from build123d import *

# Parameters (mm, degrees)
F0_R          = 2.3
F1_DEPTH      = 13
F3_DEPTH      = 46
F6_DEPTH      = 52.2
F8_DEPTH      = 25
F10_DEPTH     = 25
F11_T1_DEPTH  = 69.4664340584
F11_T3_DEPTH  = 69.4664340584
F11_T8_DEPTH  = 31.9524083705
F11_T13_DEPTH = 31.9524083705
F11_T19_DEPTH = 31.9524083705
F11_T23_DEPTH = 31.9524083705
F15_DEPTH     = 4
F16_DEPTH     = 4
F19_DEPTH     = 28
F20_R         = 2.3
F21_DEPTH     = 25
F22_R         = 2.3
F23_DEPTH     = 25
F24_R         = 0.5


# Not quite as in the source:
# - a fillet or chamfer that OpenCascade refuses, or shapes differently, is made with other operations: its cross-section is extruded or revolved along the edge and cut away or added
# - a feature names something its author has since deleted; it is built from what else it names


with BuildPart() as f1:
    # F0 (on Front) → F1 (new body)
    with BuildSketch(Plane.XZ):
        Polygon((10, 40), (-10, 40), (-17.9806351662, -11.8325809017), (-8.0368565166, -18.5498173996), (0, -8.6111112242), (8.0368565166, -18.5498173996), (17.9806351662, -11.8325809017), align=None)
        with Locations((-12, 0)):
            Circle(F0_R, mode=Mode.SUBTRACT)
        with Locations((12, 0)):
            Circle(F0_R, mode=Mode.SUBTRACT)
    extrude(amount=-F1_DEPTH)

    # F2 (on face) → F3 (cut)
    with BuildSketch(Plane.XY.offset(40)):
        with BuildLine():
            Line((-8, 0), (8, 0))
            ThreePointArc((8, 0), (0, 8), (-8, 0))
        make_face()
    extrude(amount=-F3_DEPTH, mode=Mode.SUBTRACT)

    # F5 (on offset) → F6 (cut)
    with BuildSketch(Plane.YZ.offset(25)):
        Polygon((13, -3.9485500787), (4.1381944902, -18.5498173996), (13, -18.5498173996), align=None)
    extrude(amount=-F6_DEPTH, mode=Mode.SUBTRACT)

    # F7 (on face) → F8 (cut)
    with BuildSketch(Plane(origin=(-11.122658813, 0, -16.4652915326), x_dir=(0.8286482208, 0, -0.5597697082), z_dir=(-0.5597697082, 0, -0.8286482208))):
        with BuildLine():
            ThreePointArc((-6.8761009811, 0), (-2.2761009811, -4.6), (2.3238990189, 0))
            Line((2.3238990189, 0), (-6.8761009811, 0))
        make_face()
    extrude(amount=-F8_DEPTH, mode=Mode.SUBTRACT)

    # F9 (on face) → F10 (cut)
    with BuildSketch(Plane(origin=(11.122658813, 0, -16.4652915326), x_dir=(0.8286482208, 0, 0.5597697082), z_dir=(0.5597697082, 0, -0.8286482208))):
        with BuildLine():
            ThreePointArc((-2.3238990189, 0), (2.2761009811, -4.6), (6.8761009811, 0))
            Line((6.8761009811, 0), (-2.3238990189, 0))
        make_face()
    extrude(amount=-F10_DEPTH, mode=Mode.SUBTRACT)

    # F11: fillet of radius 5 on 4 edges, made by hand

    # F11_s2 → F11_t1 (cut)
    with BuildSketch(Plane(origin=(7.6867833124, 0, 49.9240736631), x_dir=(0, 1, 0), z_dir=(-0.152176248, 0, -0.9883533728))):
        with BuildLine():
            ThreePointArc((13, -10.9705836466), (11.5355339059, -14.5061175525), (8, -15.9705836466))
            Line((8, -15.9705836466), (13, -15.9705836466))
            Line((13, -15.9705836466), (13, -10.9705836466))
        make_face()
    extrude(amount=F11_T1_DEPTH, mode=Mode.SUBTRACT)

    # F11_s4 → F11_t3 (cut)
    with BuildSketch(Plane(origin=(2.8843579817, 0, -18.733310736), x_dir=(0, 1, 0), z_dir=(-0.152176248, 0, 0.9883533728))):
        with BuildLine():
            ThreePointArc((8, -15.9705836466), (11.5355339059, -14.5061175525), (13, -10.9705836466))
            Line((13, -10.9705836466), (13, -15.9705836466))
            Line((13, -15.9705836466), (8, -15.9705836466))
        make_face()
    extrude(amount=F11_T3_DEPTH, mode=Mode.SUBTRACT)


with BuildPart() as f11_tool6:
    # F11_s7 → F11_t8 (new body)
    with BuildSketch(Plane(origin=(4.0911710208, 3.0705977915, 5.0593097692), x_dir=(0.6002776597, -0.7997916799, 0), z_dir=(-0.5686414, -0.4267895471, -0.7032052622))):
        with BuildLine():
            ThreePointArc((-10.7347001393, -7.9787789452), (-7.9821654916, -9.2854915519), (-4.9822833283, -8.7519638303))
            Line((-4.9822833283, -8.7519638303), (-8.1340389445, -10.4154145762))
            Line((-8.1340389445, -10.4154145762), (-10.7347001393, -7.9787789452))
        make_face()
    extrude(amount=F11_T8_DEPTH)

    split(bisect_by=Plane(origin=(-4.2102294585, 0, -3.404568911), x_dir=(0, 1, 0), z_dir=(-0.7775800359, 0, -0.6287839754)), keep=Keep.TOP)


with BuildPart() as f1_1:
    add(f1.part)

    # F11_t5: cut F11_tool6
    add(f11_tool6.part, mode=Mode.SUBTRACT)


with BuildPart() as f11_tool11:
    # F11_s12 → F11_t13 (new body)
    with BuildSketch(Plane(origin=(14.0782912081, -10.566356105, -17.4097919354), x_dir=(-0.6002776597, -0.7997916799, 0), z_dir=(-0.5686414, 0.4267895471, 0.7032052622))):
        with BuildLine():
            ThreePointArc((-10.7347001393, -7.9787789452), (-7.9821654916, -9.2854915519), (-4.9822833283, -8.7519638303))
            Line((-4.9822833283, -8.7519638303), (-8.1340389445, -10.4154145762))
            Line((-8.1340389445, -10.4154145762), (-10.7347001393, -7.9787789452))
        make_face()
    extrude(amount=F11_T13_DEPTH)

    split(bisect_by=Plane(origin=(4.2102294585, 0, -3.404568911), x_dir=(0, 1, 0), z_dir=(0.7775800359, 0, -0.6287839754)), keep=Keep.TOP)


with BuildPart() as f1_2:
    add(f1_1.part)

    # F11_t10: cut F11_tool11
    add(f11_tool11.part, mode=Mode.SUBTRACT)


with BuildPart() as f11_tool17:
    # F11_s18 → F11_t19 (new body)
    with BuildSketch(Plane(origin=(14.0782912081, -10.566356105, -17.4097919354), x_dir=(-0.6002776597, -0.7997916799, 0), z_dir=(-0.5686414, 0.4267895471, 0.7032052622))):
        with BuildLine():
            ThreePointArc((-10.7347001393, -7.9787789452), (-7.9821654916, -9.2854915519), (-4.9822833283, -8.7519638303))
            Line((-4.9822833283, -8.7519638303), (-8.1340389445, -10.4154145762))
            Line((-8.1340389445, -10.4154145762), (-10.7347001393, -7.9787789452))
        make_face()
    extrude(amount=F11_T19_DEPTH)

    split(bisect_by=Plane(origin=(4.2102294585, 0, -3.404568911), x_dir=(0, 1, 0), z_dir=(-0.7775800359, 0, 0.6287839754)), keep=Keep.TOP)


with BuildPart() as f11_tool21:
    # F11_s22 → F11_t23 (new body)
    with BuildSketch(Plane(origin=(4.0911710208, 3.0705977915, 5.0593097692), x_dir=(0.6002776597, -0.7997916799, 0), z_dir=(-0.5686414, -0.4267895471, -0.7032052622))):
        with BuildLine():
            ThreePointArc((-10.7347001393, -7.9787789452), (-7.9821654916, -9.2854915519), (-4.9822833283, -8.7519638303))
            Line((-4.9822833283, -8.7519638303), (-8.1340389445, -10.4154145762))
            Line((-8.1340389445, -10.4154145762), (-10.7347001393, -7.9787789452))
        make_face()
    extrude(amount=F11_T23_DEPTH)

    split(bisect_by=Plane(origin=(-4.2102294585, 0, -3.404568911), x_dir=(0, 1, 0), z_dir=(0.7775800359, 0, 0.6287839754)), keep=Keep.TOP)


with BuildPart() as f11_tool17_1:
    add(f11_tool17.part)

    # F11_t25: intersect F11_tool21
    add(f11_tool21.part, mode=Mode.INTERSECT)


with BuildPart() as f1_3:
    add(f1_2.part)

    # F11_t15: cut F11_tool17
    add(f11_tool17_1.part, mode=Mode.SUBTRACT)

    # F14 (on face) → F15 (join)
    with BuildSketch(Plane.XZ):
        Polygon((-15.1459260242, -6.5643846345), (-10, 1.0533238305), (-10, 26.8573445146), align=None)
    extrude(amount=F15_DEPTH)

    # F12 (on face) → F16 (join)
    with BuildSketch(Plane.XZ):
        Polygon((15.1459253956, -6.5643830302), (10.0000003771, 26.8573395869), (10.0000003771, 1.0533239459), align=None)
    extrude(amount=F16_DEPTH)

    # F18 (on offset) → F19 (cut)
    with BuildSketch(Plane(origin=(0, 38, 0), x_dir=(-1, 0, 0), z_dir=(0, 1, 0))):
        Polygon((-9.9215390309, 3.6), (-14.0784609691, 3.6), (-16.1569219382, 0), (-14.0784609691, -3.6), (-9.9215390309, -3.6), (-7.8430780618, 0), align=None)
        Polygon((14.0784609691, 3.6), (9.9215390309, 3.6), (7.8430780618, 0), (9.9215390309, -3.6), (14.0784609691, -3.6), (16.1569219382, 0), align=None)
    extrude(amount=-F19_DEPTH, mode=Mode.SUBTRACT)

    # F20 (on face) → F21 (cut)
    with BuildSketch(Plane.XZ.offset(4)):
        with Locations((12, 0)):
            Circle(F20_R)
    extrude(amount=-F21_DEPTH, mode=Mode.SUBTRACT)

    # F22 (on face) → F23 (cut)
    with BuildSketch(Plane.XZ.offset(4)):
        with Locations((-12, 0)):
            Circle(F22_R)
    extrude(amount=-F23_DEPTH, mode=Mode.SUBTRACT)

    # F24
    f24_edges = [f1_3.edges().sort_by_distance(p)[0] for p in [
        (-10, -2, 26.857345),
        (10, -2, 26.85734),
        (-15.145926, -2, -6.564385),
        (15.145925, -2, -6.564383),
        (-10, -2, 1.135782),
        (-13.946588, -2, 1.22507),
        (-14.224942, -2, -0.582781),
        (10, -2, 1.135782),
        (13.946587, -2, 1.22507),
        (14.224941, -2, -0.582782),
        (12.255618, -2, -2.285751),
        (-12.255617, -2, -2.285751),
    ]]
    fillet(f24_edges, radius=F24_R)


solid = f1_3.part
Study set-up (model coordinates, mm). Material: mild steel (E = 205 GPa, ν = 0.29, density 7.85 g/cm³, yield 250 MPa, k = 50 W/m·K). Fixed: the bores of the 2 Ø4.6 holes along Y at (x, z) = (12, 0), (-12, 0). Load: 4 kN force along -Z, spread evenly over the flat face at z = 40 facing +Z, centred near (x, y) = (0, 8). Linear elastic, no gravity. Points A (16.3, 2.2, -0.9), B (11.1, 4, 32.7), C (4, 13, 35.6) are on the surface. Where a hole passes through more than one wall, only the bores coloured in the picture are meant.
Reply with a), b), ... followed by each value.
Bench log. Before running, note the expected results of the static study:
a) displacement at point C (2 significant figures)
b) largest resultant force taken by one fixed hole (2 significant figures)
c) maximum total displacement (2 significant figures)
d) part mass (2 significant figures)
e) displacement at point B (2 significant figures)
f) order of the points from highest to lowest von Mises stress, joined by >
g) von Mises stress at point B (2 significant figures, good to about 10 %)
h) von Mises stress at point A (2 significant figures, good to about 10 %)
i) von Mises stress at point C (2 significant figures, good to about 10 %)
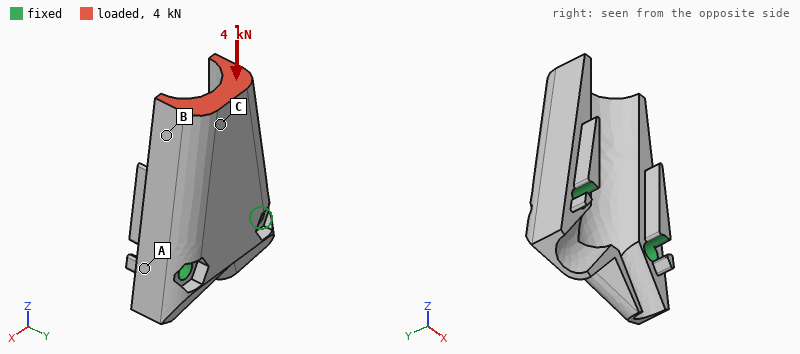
a) 8.1 µm
b) 2.0 kN
c) 9.4 µm
d) 99 g
e) 5.4 µm
f) C > B > A
g) 17 MPa
h) 5.9 MPa
i) 27 MPa
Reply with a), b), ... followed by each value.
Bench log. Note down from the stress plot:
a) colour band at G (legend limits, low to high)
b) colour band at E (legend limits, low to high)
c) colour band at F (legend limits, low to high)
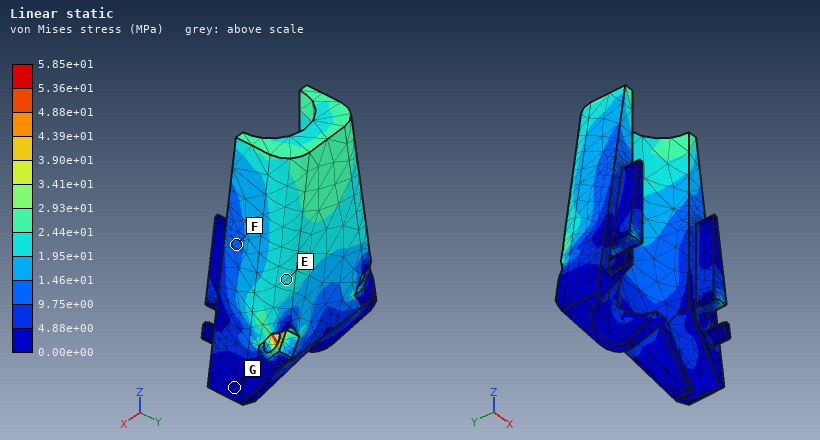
a) 0.00e+00 to 4.88e+00 MPa
b) 1.95e+01 to 2.44e+01 MPa
c) 9.75e+00 to 1.46e+01 MPa
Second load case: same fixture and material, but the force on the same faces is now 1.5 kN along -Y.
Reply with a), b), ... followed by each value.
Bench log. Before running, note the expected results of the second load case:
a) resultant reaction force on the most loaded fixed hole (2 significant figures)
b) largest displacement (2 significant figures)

a) 770 N
b) 49 µm
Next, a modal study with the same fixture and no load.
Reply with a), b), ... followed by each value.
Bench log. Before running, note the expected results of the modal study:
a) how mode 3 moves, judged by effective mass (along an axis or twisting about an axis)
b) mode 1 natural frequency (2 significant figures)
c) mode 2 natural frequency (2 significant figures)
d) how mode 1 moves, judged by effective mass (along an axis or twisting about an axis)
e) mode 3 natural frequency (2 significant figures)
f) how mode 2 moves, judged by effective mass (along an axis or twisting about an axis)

a) along X
b) 7600 Hz
c) 11 kHz
d) along Y
e) 18 kHz
f) along X
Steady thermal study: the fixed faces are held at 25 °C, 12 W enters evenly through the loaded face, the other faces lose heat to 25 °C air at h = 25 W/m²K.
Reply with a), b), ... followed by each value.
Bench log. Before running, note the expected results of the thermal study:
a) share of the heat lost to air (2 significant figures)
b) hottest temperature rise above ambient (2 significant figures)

a) 12 %
b) 41 K
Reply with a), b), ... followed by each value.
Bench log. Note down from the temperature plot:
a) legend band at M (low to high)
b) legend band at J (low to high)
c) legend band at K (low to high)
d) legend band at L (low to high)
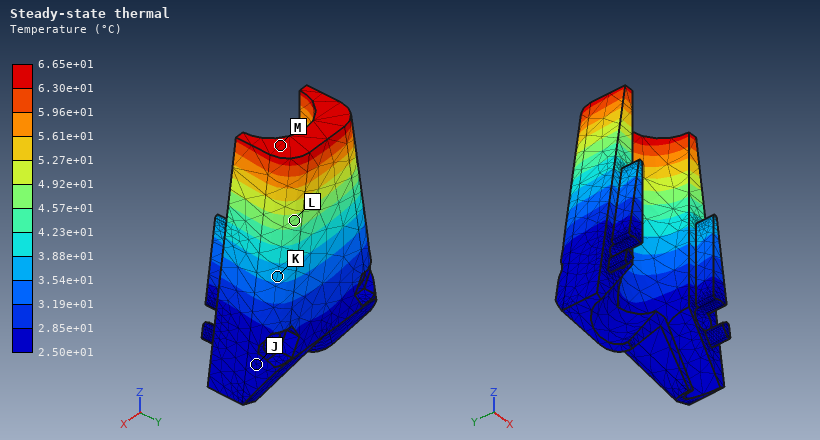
a) 6.30e+01 to 6.65e+01 °C
b) 2.50e+01 to 2.85e+01 °C
c) 3.54e+01 to 3.88e+01 °C
d) 4.57e+01 to 4.92e+01 °C
